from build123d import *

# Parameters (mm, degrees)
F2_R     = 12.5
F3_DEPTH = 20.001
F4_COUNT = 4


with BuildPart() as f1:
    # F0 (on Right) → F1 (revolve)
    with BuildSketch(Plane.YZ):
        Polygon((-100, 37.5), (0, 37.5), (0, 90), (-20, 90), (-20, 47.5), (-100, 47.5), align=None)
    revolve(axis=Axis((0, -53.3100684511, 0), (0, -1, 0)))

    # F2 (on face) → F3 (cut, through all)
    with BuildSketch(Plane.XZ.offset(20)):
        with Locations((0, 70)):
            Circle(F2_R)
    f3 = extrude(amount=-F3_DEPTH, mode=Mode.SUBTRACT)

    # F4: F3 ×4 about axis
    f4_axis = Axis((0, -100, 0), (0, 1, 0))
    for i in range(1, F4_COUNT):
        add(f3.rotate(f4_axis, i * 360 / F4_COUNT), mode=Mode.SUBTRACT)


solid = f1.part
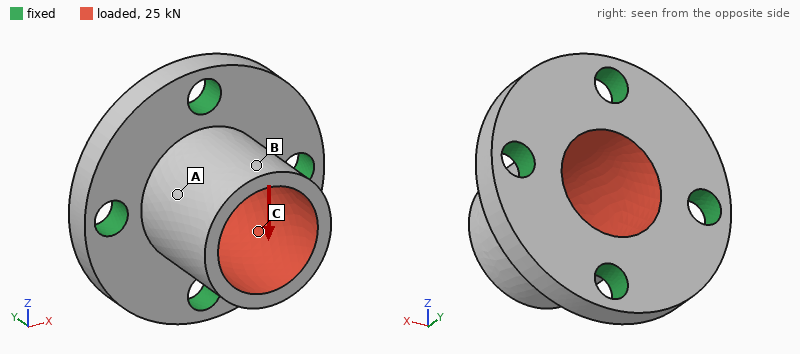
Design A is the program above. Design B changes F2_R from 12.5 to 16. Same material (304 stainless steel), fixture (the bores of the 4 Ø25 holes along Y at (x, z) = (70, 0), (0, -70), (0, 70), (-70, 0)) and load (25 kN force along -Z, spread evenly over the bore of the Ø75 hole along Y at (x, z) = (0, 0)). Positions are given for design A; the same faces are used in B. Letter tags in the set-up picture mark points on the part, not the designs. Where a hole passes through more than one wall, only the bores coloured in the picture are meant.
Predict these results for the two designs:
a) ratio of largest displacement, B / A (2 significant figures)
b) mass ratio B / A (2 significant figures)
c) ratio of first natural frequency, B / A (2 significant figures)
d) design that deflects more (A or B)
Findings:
0.90
0.96
1.0
A
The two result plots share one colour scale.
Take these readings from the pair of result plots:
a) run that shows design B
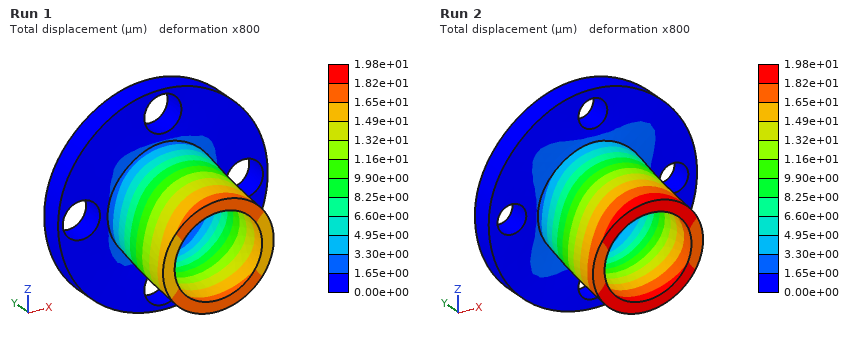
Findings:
Run 1
